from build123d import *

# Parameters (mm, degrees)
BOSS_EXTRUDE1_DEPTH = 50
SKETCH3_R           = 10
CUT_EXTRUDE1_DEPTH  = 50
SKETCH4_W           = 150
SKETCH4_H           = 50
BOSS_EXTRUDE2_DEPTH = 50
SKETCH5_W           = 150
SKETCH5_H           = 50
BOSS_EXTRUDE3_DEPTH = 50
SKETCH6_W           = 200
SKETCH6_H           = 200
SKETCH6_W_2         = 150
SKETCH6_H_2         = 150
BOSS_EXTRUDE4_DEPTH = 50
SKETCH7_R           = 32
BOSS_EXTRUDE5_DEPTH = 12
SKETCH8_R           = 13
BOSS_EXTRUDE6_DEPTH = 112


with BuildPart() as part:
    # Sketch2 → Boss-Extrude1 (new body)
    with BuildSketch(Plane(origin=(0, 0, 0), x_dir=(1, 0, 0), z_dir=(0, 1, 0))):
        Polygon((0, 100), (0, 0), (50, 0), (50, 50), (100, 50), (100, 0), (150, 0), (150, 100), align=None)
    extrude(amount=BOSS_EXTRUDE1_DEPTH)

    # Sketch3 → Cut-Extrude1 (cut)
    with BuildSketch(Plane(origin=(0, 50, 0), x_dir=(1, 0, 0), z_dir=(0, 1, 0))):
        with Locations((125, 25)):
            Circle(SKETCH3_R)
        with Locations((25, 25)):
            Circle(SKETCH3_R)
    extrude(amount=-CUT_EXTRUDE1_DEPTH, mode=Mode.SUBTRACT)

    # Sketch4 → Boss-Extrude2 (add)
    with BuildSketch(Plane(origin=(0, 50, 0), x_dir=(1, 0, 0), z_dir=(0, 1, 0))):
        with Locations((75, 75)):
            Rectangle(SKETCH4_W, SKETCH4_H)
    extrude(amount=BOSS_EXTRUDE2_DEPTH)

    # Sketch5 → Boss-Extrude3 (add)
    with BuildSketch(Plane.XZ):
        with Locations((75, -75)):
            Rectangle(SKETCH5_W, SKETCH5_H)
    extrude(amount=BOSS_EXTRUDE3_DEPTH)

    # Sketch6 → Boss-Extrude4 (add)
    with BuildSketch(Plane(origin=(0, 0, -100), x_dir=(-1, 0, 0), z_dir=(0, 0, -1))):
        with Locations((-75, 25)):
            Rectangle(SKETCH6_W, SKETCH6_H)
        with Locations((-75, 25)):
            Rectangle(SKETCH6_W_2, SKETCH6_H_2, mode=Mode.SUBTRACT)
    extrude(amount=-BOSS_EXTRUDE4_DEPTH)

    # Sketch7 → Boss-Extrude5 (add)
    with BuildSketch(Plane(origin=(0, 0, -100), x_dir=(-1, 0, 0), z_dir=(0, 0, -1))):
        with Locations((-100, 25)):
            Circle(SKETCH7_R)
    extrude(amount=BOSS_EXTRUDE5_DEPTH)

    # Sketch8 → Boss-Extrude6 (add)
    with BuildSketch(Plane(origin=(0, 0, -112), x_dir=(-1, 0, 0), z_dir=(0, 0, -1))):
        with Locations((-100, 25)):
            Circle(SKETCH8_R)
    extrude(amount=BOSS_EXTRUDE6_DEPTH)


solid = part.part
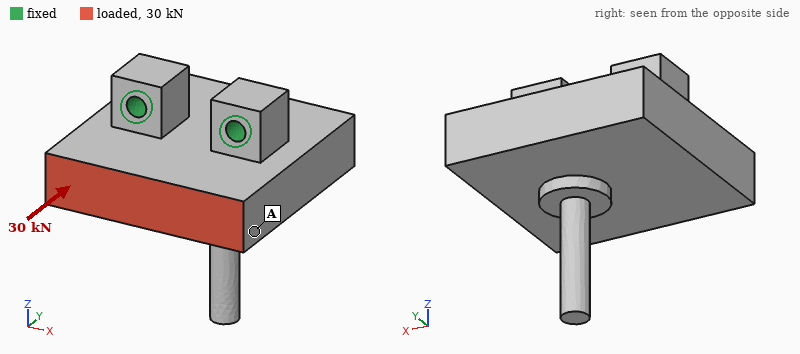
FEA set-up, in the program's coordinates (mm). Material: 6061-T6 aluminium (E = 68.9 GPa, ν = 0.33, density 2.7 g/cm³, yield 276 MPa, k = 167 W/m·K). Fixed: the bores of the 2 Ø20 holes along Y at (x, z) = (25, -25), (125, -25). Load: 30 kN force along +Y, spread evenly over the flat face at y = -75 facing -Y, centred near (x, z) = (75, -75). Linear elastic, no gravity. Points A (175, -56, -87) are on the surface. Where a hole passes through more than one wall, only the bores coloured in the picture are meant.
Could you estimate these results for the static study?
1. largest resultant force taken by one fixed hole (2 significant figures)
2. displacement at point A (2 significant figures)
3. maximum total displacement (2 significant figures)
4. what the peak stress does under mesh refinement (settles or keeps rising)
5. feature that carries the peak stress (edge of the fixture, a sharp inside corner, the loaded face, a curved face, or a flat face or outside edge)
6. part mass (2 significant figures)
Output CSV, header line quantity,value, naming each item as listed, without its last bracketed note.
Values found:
quantity,value
largest resultant force taken by one fixed hole,15 kN
displacement at point A,50 µm
maximum total displacement,91 µm
what the peak stress does under mesh refinement,keeps rising
feature that carries the peak stress,edge of the fixture
part mass,6.3 kg
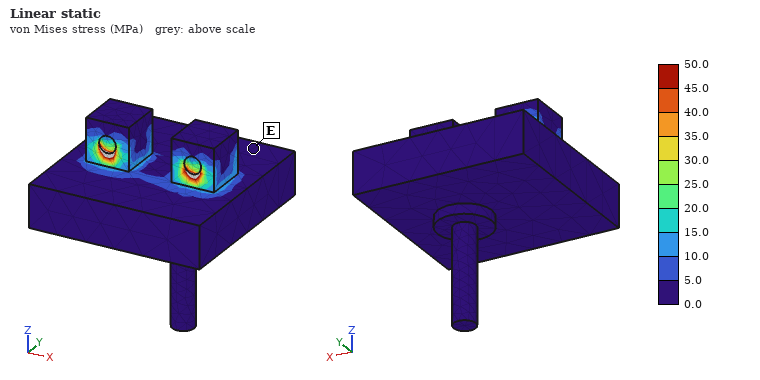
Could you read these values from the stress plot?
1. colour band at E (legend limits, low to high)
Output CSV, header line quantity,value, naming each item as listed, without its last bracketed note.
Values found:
quantity,value
colour band at E,0.0 to 5.0 MPa
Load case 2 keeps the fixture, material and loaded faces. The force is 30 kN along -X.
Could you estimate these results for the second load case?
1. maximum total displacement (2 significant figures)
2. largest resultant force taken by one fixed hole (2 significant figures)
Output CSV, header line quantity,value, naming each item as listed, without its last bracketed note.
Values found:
quantity,value
maximum total displacement,78 µm
largest resultant force taken by one fixed hole,30 kN
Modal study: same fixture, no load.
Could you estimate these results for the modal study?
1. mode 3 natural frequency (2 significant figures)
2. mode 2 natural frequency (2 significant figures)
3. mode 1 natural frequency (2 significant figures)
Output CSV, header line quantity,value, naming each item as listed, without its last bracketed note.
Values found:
quantity,value
mode 3 natural frequency,1500 Hz
mode 2 natural frequency,1300 Hz
mode 1 natural frequency,1200 Hz
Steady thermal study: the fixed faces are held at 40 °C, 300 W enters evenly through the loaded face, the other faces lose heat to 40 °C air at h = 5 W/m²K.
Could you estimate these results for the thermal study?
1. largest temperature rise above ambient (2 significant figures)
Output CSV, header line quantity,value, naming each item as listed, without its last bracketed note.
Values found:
quantity,value
largest temperature rise above ambient,27 K
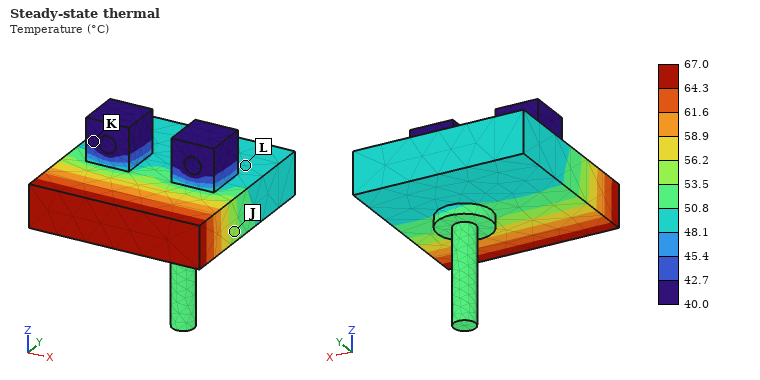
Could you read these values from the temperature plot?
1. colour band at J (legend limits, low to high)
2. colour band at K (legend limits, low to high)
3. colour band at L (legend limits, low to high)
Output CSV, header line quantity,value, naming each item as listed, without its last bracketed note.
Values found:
quantity,value
colour band at J,53.5 to 56.2 °C
colour band at K,40.0 to 42.7 °C
colour band at L,48.1 to 50.8 °C
